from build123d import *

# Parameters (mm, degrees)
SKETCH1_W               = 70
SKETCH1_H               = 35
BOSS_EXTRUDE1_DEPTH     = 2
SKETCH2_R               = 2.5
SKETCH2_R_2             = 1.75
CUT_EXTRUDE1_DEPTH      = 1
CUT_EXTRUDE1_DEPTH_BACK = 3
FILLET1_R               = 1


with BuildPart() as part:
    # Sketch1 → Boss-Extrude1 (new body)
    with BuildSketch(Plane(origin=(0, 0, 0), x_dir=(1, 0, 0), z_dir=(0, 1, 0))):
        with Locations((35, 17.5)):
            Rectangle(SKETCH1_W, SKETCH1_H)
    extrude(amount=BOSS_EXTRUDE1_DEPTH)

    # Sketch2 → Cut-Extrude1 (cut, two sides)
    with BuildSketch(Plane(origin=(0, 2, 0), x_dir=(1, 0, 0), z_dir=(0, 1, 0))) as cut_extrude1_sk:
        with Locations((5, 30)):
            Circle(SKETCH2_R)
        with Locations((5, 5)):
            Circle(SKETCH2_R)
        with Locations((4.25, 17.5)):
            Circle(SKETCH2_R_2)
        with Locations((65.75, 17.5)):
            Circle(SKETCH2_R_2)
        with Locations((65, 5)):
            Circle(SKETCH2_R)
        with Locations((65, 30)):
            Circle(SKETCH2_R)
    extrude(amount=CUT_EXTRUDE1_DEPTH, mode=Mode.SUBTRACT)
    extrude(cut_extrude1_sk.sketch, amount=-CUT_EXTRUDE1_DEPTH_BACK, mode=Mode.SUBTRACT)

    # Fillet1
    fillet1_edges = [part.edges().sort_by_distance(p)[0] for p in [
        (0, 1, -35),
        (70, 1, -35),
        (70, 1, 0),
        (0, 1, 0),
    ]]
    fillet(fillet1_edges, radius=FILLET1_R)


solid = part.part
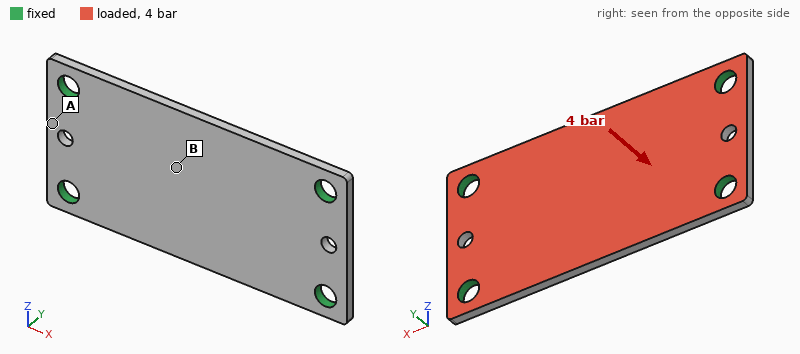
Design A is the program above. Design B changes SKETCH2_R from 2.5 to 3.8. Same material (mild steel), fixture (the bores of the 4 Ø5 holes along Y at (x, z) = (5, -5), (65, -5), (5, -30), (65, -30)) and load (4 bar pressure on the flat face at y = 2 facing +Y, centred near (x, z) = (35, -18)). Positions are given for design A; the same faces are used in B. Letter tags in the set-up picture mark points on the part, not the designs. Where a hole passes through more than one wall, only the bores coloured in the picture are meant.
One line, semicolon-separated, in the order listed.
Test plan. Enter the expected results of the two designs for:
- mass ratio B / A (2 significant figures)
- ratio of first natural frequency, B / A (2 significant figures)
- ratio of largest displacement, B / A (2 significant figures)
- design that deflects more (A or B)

0.96; 1.1; 0.80; A
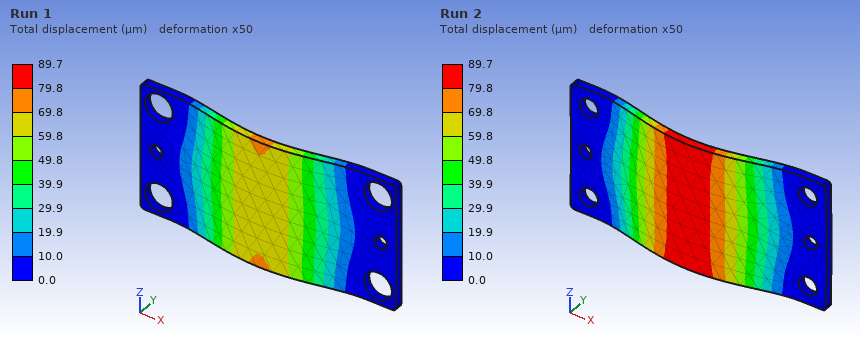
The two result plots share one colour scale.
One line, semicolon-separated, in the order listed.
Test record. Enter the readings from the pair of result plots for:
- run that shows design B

Run 1
